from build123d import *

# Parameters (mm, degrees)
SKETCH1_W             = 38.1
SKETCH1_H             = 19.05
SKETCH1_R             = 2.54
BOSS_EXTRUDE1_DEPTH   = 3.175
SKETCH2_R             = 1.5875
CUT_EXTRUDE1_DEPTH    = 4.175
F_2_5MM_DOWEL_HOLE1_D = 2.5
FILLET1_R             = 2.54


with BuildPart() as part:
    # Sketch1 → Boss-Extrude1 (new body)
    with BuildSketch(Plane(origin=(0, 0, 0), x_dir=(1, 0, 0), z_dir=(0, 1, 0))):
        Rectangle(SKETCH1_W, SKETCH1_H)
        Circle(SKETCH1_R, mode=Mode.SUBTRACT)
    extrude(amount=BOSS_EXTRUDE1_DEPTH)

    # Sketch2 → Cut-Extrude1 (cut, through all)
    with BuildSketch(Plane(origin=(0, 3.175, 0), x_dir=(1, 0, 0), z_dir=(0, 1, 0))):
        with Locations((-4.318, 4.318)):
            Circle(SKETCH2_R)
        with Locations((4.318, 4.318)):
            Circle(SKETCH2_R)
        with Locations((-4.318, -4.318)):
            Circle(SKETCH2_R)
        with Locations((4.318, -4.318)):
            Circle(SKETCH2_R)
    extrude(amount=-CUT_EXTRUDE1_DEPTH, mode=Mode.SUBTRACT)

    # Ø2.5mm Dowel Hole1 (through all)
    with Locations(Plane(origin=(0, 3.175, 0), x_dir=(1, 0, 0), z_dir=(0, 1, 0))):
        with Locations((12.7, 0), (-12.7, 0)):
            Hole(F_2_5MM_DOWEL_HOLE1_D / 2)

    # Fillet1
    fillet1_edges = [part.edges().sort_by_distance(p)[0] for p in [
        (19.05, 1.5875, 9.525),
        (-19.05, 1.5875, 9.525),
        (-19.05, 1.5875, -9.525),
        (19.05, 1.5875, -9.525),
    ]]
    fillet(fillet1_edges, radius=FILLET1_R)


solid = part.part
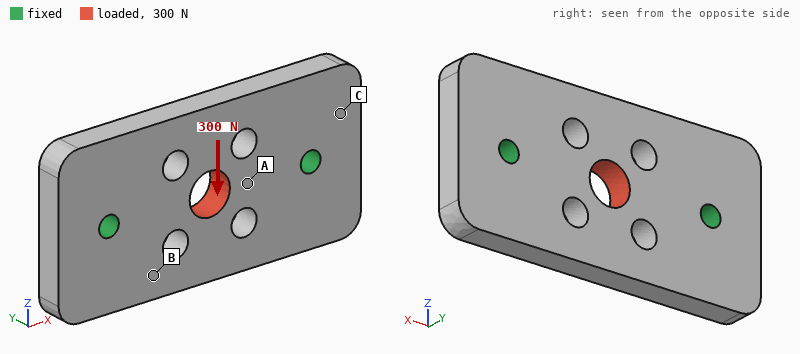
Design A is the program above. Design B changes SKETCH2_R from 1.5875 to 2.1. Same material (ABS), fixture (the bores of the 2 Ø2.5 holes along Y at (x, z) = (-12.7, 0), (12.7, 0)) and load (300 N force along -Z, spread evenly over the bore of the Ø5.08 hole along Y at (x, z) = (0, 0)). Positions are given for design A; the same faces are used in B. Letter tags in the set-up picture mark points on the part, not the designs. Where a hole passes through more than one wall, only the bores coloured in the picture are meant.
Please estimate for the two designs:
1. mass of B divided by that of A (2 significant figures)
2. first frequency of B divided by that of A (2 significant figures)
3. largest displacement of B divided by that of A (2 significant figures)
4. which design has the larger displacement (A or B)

0.96
1.0
1.2
B
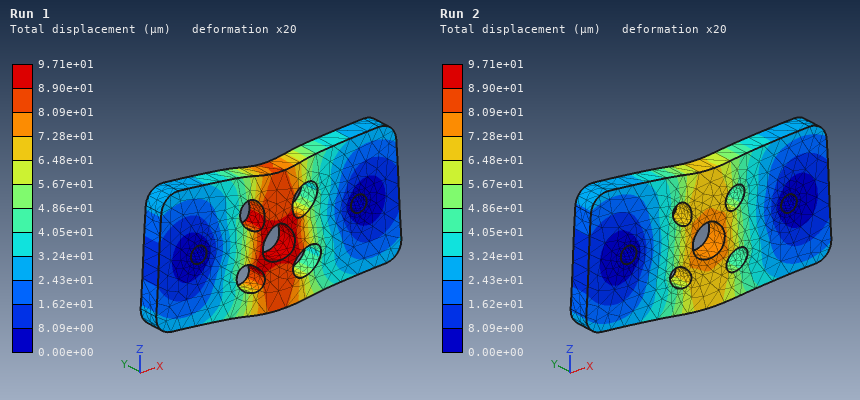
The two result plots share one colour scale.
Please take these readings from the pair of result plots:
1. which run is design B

Run 1
